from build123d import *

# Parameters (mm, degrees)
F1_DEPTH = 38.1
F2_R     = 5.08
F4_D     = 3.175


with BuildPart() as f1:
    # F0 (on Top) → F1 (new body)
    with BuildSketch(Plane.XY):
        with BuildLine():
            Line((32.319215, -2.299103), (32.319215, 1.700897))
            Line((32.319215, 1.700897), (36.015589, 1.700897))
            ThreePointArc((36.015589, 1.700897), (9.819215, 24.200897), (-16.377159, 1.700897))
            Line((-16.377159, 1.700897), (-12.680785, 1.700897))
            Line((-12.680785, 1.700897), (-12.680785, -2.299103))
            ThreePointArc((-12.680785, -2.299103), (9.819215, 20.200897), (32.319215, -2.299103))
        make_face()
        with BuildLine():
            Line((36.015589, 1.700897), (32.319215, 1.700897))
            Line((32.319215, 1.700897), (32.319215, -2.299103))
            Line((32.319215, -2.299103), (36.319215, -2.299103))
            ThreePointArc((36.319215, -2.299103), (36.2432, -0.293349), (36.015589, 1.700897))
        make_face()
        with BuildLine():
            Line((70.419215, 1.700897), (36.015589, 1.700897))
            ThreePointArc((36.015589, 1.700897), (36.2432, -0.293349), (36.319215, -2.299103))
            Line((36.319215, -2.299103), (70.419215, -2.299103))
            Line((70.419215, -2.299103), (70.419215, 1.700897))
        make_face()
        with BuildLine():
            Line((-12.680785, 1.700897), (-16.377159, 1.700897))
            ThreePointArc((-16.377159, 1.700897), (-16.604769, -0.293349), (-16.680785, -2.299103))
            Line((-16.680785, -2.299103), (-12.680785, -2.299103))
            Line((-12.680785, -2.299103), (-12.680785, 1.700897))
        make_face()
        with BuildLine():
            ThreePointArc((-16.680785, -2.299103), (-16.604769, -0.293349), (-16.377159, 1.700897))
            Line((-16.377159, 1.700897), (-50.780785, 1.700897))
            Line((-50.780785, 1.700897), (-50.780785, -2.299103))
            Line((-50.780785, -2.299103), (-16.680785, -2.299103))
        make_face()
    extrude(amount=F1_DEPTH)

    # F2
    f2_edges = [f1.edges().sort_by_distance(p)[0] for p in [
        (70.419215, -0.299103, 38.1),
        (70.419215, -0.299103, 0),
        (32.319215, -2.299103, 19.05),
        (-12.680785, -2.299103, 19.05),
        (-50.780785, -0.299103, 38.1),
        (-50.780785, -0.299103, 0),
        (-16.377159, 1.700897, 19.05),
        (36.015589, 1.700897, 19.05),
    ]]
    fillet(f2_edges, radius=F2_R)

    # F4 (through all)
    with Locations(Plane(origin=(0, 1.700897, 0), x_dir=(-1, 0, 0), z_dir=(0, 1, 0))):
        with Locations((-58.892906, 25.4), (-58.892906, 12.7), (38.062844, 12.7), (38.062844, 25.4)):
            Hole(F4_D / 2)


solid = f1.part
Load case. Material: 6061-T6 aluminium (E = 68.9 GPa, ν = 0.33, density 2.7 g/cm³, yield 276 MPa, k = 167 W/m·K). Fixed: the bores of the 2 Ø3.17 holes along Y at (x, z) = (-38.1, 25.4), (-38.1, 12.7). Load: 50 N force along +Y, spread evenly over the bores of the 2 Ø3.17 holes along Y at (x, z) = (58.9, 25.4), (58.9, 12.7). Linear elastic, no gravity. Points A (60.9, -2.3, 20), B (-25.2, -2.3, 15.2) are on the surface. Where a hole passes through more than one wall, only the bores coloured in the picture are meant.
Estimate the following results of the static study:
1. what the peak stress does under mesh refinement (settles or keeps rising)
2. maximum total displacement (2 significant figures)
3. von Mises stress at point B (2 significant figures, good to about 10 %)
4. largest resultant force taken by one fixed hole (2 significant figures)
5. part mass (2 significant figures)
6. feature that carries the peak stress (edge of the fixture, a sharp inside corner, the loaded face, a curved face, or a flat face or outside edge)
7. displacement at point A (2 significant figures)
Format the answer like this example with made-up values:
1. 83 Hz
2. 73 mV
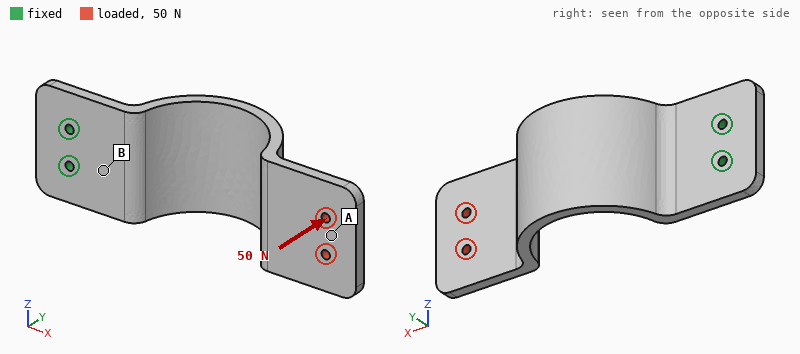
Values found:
1. keeps rising
2. 1.4 mm
3. 37 MPa
4. 30 N
5. 59 g
6. edge of the fixture
7. 1.3 mm
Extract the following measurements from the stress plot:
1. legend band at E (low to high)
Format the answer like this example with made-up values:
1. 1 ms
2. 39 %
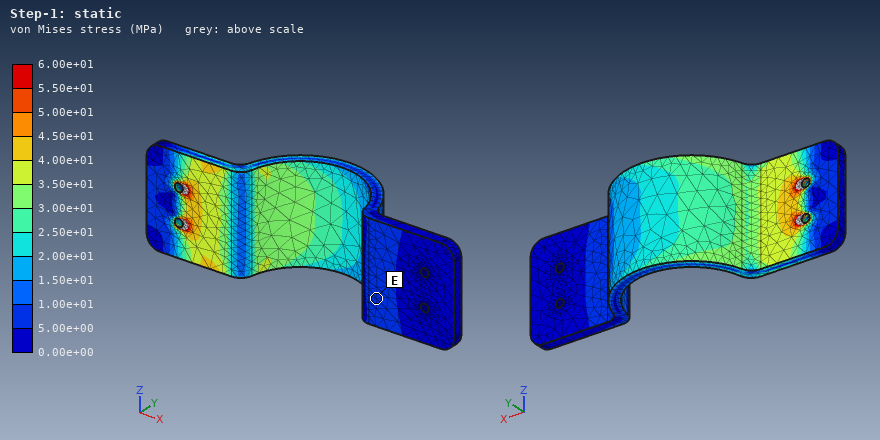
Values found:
1. 5.00e+00 to 1.00e+01 MPa
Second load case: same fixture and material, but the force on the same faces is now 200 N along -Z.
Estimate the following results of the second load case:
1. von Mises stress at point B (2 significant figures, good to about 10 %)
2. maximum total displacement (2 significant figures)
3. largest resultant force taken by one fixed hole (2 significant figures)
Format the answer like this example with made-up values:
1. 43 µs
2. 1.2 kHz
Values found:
1. 30 MPa
2. 1.1 mm
3. 1.3 kN
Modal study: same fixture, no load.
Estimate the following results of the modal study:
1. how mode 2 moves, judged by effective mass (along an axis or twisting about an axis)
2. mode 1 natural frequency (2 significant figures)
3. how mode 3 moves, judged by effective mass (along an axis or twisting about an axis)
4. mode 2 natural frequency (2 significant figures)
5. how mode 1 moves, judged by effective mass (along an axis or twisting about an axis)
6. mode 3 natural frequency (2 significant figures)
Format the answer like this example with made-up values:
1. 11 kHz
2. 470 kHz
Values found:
1. along Z
2. 250 Hz
3. along X
4. 570 Hz
5. along Y
6. 950 Hz
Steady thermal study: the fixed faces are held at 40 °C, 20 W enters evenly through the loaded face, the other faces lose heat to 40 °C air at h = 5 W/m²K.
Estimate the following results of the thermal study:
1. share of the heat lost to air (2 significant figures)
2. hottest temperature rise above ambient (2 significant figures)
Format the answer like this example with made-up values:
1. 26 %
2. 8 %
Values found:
1. 13 %
2. 87 K
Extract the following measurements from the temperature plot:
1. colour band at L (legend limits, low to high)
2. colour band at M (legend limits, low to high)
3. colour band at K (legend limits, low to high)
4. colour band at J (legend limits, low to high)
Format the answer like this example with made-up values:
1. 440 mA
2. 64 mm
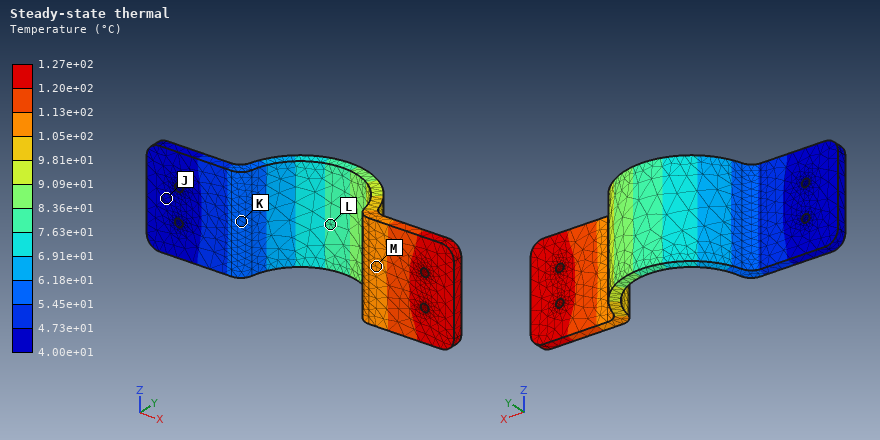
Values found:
1. 7.63e+01 to 8.36e+01 °C
2. 1.05e+02 to 1.13e+02 °C
3. 5.45e+01 to 6.18e+01 °C
4. 4.00e+01 to 4.73e+01 °C
